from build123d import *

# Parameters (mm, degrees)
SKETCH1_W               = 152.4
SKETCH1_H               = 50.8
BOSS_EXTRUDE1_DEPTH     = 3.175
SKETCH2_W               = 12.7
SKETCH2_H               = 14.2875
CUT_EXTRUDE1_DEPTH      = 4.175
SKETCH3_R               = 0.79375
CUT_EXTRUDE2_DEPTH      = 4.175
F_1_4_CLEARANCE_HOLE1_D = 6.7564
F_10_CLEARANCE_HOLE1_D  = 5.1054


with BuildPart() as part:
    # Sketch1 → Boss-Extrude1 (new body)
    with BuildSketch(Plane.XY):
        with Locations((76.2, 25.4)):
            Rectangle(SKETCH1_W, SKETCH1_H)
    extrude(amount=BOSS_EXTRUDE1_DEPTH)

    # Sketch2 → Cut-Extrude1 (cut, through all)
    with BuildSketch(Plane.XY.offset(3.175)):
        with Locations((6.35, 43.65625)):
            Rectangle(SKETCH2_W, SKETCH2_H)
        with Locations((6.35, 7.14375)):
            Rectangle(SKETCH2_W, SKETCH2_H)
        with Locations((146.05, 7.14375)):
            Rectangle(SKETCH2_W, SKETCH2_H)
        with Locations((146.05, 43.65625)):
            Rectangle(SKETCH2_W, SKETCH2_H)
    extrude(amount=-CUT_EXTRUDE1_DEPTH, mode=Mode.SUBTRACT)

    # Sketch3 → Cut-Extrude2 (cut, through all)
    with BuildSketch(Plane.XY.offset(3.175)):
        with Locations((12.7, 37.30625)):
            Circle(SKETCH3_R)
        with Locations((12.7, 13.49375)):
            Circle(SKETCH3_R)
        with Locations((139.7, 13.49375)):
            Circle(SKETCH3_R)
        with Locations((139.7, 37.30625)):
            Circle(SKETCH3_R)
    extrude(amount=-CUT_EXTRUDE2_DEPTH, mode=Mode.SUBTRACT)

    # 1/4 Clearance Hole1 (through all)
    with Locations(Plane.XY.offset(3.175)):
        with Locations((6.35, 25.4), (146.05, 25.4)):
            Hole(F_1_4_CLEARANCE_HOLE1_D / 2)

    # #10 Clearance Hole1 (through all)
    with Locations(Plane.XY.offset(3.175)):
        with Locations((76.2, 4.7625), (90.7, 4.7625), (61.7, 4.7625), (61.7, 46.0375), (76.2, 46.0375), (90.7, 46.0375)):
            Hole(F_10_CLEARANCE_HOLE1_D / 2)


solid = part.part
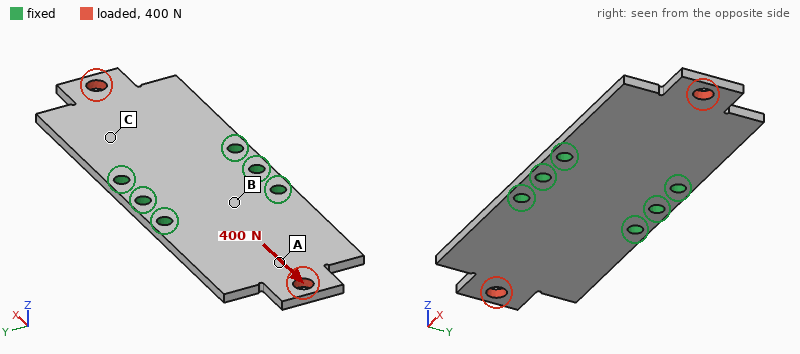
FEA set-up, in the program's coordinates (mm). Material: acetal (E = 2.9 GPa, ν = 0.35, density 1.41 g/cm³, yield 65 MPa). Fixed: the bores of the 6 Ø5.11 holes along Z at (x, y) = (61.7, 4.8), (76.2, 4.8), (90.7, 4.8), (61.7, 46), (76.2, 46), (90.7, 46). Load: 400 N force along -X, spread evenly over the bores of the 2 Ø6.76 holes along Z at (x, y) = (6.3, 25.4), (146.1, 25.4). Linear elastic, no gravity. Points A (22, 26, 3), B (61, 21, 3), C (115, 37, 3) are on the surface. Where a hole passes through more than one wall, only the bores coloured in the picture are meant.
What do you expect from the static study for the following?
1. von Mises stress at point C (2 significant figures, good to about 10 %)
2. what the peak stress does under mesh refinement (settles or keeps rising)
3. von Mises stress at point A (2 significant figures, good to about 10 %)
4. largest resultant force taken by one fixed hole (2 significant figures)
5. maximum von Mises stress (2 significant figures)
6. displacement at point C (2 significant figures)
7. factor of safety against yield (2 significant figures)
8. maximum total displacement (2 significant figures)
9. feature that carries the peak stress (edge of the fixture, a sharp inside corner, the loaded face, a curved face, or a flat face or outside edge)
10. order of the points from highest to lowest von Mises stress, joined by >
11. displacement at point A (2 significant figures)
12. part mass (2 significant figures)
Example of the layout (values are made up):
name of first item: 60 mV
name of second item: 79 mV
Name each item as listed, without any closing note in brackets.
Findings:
von Mises stress at point C: 1.5 MPa
what the peak stress does under mesh refinement: settles
von Mises stress at point A: 2.3 MPa
largest resultant force taken by one fixed hole: 85 N
maximum von Mises stress: 9.5 MPa
displacement at point C: 14 µm
factor of safety against yield: 6.8
maximum total displacement: 57 µm
feature that carries the peak stress: the loaded face
order of the points from highest to lowest von Mises stress, joined by >: A > C > B
displacement at point A: 25 µm
part mass: 31 g
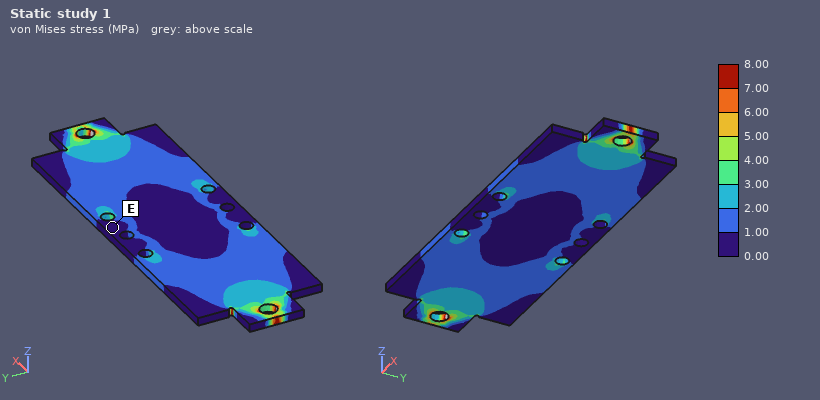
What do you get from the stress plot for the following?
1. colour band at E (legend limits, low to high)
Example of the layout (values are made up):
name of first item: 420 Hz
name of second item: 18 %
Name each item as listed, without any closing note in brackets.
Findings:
colour band at E: 0.00 to 1.00 MPa
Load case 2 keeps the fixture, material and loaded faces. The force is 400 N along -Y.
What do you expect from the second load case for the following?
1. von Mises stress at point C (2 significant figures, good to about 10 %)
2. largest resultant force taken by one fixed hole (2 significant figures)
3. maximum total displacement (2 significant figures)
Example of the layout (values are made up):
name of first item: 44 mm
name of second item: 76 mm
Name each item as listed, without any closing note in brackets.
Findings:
von Mises stress at point C: 3.5 MPa
largest resultant force taken by one fixed hole: 250 N
maximum total displacement: 0.26 mm
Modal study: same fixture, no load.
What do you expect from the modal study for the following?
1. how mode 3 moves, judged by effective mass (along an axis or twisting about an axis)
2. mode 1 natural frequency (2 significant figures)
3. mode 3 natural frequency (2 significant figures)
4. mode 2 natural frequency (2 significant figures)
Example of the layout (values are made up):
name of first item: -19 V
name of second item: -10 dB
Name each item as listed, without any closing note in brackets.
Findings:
how mode 3 moves, judged by effective mass: twisting about X
mode 1 natural frequency: 240 Hz
mode 3 natural frequency: 730 Hz
mode 2 natural frequency: 240 Hz
